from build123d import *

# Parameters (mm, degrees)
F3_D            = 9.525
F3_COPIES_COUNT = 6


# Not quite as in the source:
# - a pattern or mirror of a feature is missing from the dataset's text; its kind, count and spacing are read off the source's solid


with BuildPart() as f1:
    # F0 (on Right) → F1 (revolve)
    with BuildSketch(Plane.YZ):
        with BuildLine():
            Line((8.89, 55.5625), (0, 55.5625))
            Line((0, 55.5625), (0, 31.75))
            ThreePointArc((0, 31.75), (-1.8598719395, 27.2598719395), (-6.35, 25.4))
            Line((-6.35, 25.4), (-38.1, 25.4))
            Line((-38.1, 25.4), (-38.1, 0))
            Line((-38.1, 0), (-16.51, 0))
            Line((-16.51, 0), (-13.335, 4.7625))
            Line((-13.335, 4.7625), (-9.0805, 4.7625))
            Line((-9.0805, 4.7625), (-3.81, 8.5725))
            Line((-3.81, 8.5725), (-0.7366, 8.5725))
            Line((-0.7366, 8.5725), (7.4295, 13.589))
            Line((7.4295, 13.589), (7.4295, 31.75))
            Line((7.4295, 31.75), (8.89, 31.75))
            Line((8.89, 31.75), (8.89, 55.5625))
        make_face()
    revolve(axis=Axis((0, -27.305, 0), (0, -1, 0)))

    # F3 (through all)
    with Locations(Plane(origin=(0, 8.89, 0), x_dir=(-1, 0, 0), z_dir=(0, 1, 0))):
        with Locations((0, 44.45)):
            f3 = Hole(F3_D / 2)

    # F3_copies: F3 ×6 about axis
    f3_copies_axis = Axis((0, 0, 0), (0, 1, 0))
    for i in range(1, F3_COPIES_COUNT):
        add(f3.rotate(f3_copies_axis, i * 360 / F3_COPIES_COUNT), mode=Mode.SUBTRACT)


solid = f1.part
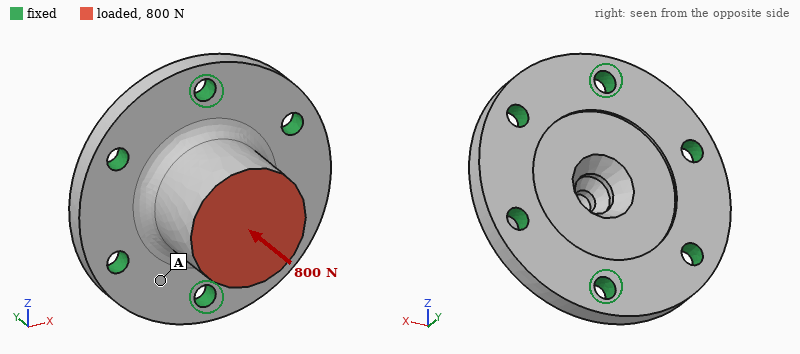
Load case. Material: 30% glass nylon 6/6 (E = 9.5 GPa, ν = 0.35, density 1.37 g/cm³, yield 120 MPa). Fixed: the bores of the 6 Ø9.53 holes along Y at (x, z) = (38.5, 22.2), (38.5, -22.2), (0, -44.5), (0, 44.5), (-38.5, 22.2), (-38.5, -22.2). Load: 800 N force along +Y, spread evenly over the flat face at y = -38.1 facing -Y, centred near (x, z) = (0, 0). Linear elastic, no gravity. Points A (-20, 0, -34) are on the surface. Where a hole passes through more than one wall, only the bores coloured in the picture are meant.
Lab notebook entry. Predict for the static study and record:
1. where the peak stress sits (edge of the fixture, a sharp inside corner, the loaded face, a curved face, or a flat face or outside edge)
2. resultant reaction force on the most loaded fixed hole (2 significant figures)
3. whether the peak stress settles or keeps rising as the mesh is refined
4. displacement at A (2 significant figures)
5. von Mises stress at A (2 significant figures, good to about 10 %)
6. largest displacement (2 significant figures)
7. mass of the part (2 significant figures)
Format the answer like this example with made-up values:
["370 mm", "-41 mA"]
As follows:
["edge of the fixture", "160 N", "keeps rising", "2.8 µm", "0.69 MPa", "10 µm", "210 g"]
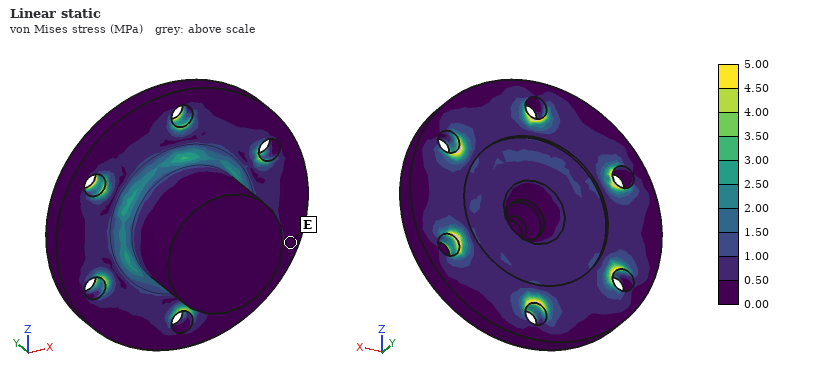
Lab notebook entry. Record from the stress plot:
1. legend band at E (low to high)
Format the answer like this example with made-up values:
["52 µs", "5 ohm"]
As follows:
["0.00 to 0.50 MPa"]
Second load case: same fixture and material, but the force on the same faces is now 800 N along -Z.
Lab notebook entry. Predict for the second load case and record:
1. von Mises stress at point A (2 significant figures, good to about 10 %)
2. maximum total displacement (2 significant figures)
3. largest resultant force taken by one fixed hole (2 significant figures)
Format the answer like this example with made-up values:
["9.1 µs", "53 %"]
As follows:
["1.3 MPa", "38 µm", "390 N"]
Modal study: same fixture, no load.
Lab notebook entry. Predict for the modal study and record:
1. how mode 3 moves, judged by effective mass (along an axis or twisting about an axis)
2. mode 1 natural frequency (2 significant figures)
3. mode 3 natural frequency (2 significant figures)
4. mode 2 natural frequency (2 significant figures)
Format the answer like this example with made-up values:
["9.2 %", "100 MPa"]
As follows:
["along Y", "3700 Hz", "4100 Hz", "3700 Hz"]
